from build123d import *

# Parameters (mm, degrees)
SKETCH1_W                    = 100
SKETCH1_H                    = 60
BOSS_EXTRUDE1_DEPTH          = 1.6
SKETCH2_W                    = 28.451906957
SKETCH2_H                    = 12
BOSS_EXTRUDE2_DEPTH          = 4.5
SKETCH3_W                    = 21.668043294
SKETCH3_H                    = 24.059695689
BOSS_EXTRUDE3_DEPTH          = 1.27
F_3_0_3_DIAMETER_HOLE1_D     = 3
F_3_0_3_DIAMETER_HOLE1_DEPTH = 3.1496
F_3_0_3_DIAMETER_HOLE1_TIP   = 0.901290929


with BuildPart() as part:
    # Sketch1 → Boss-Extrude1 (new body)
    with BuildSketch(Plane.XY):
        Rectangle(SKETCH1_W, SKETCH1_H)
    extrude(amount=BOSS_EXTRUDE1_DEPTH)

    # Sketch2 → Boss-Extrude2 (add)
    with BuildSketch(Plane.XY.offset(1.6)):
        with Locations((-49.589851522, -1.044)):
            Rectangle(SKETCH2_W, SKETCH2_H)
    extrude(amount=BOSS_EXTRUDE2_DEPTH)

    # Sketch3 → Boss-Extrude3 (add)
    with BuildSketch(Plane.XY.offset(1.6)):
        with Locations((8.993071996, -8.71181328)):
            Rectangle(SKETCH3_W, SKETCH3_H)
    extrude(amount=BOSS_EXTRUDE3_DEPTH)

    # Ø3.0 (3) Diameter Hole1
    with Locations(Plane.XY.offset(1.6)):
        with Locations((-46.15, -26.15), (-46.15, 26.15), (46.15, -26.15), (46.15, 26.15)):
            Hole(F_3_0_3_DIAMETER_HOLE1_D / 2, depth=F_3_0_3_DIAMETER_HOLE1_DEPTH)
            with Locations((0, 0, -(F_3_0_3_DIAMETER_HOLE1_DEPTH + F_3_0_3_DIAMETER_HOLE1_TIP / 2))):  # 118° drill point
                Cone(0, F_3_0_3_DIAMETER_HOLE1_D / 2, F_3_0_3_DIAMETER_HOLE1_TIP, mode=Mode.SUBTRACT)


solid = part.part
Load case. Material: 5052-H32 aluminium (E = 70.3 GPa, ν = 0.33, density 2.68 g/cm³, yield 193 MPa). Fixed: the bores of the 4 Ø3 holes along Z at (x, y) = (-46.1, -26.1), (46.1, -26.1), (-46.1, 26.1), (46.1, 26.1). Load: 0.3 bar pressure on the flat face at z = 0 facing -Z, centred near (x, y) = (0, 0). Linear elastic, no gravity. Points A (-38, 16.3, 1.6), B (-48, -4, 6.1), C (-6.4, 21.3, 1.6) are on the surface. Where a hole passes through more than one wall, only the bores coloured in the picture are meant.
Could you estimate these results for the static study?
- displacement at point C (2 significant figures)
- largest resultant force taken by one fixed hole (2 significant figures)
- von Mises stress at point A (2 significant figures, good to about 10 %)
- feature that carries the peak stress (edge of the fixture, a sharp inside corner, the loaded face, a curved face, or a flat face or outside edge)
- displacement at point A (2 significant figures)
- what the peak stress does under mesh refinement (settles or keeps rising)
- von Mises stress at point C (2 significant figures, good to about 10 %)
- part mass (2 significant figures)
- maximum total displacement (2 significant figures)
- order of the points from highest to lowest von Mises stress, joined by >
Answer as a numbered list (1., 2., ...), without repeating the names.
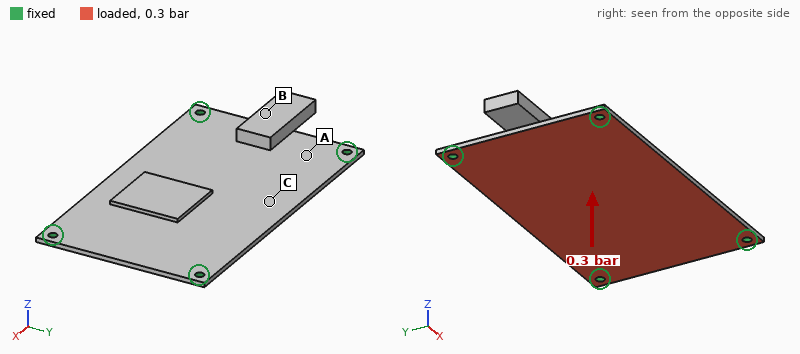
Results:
1. 0.29 mm
2. 54 N
3. 16 MPa
4. edge of the fixture
5. 0.065 mm
6. keeps rising
7. 27 MPa
8. 31 g
9. 0.31 mm
10. C > A > B
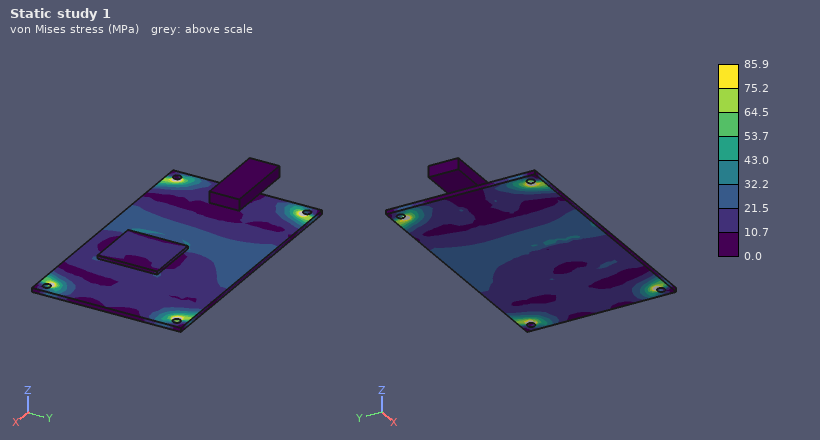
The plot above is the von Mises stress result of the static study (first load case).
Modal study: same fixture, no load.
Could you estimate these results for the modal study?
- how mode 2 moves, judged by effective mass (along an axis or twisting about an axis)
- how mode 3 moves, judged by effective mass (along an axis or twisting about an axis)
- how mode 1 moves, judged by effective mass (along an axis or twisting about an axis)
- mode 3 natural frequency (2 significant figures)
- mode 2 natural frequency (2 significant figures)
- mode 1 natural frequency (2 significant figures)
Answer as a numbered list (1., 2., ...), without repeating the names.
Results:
1. twisting about X
2. along Z
3. along Z
4. 1800 Hz
5. 1500 Hz
6. 830 Hz
